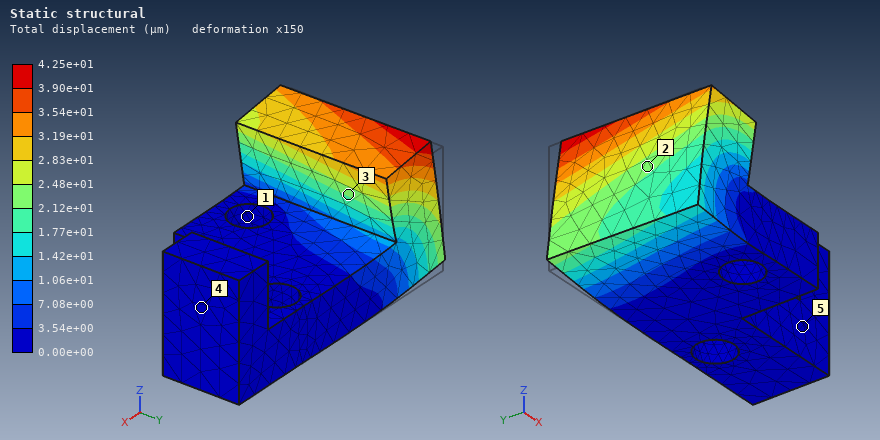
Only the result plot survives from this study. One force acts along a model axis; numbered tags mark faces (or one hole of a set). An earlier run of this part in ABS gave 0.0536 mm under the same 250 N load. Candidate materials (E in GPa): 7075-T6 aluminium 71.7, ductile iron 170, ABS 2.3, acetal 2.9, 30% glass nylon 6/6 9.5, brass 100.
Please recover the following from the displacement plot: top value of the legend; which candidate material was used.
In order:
4.25e+01 µm
acetal
